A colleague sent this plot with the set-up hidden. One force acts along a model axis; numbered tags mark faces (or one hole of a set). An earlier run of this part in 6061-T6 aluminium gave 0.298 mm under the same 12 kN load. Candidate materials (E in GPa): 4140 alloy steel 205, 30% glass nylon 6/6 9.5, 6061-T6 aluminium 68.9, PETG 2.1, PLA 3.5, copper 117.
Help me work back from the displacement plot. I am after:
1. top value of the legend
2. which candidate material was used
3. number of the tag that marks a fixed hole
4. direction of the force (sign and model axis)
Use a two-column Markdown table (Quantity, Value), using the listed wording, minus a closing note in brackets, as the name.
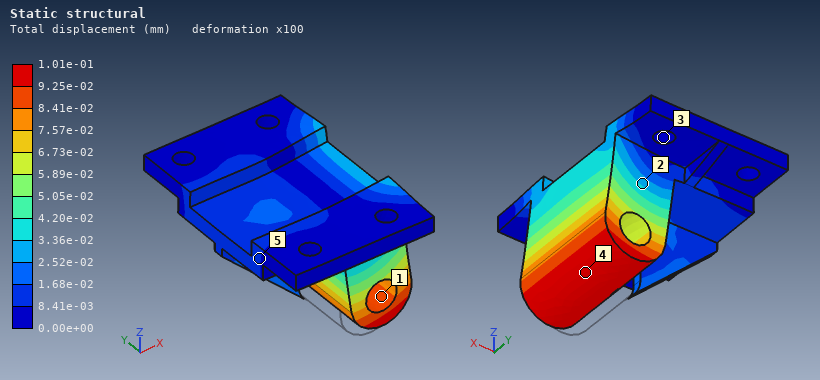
| Quantity | Value |
|---|---|
| top value of the legend | 1.01e-01 mm |
| which candidate material was used | 4140 alloy steel |
| number of the tag that marks a fixed hole | 3 |
| direction of the force | +X |
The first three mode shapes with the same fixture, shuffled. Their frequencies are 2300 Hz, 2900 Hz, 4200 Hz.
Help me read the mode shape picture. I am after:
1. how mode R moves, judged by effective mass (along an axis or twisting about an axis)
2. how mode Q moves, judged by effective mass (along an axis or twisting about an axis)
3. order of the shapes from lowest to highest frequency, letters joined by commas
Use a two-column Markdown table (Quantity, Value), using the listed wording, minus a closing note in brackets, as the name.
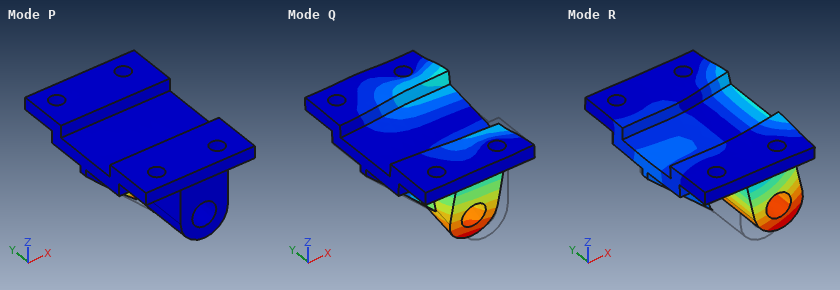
| Quantity | Value |
|---|---|
| how mode R moves, judged by effective mass | along X |
| how mode Q moves, judged by effective mass | along Y |
| order of the shapes from lowest to highest frequency, letters joined by commas | R, P, Q |
